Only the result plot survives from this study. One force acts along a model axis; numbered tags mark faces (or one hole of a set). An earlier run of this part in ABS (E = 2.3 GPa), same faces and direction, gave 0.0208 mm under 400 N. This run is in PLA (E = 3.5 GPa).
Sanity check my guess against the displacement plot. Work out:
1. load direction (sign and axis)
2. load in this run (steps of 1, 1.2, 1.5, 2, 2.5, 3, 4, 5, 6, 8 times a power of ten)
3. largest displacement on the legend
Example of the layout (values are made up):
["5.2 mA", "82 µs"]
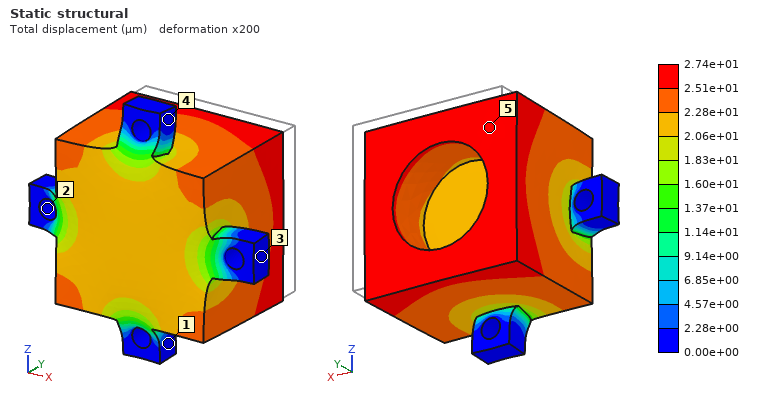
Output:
["-Y", "800 N", "2.74e+01 µm"]
